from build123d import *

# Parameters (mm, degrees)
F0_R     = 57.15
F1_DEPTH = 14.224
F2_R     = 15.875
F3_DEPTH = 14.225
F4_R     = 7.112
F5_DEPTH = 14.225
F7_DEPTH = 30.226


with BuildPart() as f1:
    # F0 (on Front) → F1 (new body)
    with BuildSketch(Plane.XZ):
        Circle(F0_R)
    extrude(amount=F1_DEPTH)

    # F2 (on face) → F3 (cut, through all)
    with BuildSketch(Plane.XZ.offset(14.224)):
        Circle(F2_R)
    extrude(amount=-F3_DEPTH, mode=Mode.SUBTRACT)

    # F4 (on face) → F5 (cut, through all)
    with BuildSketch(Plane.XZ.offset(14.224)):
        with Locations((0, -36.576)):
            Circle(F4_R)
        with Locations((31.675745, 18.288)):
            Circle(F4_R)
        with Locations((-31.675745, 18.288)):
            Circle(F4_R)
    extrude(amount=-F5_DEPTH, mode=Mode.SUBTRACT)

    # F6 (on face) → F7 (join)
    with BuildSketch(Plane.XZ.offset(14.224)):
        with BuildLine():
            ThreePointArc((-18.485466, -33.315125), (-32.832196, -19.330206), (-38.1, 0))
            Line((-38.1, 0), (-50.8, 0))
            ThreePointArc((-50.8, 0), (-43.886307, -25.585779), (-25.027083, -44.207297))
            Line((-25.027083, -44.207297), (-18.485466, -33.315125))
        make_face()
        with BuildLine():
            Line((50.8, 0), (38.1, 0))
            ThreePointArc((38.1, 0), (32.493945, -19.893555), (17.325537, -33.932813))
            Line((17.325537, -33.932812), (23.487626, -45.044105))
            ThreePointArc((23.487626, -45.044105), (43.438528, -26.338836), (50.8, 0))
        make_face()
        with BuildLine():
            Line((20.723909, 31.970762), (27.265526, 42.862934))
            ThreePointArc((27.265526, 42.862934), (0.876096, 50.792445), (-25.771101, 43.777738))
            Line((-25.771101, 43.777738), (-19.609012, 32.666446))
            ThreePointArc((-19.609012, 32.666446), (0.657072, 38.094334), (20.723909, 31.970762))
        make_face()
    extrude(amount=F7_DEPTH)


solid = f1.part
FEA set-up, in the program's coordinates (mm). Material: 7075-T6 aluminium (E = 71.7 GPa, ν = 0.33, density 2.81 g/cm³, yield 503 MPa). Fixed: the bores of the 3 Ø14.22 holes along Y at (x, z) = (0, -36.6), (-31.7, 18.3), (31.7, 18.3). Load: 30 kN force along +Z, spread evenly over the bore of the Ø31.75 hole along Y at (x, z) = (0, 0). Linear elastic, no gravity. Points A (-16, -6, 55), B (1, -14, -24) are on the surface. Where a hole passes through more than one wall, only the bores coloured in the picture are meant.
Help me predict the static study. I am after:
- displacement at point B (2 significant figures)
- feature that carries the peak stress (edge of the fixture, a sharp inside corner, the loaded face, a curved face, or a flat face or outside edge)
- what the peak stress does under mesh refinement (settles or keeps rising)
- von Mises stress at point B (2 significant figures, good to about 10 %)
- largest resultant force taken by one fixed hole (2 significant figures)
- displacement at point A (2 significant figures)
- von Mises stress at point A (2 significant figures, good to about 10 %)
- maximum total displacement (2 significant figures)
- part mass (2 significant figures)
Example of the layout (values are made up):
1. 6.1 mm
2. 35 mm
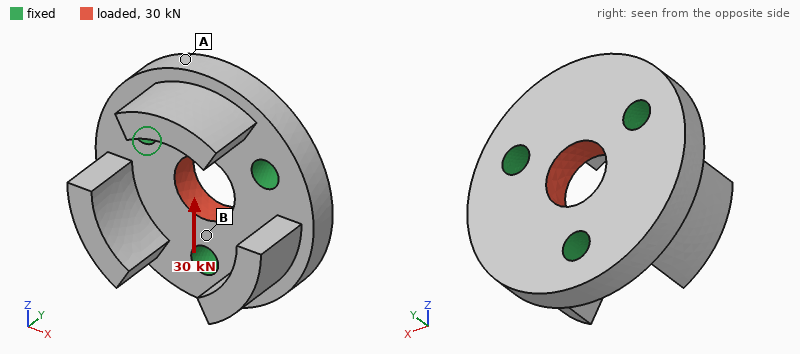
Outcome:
1. 2.4 µm
2. edge of the fixture
3. keeps rising
4. 28 MPa
5. 10 kN
6. 5.5 µm
7. 9.0 MPa
8. 13 µm
9. 520 g
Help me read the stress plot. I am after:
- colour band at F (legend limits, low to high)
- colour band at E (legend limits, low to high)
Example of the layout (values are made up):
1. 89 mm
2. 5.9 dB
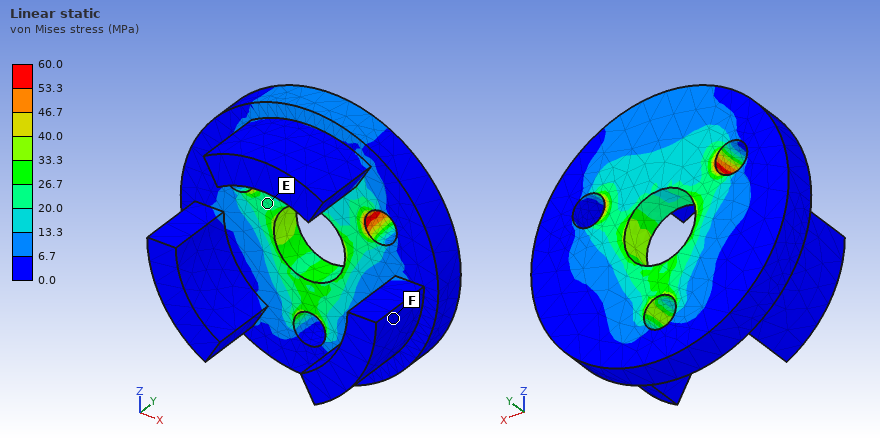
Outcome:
1. 0.0 to 6.7 MPa
2. 20.0 to 26.7 MPa
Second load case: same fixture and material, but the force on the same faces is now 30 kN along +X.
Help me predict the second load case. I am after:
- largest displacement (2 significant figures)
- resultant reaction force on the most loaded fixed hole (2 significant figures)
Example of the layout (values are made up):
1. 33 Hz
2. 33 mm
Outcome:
1. 12 µm
2. 10 kN
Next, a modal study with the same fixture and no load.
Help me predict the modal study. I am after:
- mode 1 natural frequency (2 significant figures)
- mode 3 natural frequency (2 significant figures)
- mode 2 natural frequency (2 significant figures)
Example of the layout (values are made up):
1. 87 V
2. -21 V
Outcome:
1. 4700 Hz
2. 4800 Hz
3. 4700 Hz
